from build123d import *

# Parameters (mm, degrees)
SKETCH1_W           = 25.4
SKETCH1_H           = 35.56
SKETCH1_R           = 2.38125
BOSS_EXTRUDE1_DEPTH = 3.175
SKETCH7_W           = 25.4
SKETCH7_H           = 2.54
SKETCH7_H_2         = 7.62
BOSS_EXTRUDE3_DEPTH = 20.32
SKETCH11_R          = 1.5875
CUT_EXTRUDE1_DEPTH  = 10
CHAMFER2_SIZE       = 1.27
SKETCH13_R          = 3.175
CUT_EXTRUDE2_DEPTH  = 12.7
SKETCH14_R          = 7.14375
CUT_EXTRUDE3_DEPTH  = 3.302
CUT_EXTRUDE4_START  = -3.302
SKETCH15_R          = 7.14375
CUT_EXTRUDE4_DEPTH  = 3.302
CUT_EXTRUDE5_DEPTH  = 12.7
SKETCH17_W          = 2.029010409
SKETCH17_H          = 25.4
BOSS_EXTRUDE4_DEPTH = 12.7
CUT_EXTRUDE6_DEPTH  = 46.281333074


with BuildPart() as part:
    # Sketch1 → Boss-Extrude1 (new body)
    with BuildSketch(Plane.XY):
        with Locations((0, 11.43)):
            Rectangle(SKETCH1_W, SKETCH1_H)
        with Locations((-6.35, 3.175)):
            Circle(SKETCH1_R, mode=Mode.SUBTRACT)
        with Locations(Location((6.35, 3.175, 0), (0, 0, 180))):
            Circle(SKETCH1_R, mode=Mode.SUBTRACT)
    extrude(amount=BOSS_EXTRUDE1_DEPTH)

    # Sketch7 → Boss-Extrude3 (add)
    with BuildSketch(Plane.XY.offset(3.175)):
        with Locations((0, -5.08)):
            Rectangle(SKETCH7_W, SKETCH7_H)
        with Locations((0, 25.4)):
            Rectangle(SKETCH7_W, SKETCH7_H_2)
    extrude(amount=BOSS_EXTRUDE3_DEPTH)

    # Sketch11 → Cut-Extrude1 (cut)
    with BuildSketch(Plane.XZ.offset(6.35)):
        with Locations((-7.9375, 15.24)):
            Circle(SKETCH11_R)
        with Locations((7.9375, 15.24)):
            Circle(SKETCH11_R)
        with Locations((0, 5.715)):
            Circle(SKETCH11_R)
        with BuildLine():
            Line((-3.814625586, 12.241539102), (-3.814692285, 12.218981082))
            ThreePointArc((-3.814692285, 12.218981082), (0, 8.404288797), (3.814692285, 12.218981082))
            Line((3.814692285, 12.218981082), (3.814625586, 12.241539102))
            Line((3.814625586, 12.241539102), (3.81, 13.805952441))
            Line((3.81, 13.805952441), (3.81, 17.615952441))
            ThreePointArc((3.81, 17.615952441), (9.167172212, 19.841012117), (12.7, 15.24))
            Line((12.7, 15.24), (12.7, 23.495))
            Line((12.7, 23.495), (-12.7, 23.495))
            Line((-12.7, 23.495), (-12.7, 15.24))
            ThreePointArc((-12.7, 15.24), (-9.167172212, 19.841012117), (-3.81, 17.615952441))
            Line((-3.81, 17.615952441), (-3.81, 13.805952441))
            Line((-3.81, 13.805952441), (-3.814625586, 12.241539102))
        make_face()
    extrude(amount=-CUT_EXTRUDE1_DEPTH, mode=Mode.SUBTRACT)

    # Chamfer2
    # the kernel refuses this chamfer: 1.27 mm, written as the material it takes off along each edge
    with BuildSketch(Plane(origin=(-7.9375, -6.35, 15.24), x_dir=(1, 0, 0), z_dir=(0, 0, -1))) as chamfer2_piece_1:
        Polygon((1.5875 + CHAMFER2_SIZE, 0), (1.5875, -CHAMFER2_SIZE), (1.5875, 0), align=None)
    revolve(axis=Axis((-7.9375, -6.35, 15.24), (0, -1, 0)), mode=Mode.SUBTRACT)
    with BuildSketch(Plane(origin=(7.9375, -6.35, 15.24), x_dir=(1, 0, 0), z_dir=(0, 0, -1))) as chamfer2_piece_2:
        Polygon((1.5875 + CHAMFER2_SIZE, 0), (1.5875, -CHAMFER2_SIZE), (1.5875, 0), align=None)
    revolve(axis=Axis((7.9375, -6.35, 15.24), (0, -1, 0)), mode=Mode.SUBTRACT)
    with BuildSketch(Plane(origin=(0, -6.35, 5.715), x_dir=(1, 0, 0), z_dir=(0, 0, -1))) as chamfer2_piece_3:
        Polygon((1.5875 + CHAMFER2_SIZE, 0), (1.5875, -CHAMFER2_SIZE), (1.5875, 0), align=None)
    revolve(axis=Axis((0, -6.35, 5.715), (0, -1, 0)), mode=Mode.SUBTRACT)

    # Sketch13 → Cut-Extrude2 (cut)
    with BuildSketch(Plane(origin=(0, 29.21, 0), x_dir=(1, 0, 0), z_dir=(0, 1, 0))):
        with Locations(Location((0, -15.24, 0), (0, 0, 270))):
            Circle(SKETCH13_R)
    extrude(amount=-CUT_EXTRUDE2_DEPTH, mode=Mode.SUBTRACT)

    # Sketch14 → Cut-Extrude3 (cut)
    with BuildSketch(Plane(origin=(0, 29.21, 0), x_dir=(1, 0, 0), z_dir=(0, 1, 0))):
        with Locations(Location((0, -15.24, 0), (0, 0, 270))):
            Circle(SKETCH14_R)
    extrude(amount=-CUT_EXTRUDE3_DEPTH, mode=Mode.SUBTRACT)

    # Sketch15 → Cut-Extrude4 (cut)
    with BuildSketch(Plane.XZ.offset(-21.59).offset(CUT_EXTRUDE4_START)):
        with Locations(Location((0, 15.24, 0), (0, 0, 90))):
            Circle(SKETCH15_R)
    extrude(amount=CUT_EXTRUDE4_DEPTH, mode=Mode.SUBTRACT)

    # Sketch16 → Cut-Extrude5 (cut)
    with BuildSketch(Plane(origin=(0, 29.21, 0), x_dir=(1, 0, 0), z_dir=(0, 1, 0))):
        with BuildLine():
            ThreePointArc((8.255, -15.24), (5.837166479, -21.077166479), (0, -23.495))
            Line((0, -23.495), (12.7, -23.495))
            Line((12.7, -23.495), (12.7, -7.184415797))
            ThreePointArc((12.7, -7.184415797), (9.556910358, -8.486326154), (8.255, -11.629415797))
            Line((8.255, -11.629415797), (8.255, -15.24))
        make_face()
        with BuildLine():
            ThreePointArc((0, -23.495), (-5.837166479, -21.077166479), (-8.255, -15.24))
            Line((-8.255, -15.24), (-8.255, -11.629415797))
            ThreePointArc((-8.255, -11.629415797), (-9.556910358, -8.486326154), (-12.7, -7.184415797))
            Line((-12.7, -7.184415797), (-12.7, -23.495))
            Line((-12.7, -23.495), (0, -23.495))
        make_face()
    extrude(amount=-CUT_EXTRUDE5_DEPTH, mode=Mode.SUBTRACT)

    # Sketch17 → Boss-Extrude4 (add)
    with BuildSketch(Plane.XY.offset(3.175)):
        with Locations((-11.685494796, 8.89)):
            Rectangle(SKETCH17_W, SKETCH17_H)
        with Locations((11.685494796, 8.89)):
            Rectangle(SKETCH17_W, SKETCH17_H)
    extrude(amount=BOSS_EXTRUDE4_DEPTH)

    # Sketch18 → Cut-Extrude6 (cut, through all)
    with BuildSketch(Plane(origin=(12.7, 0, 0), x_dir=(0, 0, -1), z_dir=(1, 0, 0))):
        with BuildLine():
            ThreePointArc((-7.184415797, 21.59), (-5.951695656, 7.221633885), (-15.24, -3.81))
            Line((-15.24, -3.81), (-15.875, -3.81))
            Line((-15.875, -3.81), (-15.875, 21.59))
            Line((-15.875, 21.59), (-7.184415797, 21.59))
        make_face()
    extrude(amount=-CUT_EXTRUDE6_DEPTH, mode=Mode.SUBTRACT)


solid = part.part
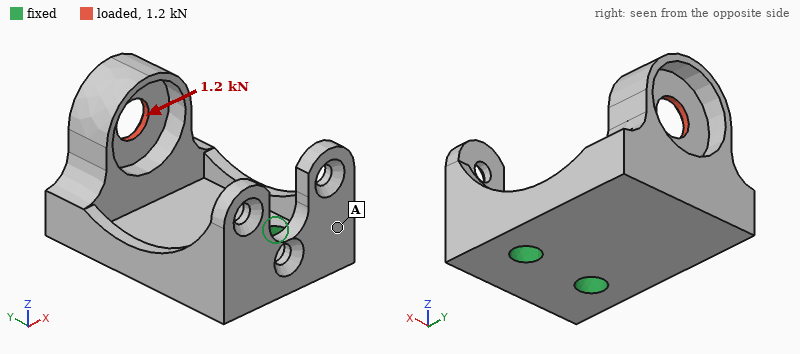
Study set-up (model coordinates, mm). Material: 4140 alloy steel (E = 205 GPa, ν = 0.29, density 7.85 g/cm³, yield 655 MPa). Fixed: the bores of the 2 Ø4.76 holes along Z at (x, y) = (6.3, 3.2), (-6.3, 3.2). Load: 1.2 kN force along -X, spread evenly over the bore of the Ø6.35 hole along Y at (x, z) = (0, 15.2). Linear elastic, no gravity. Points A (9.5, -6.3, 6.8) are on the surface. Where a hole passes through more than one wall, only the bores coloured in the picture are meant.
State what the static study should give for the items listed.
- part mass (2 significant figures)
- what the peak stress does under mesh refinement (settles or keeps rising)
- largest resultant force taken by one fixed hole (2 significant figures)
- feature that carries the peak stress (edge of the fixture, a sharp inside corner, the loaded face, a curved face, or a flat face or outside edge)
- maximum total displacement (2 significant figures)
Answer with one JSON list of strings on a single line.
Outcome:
["43 g", "keeps rising", "1.9 kN", "edge of the fixture", "0.13 mm"]
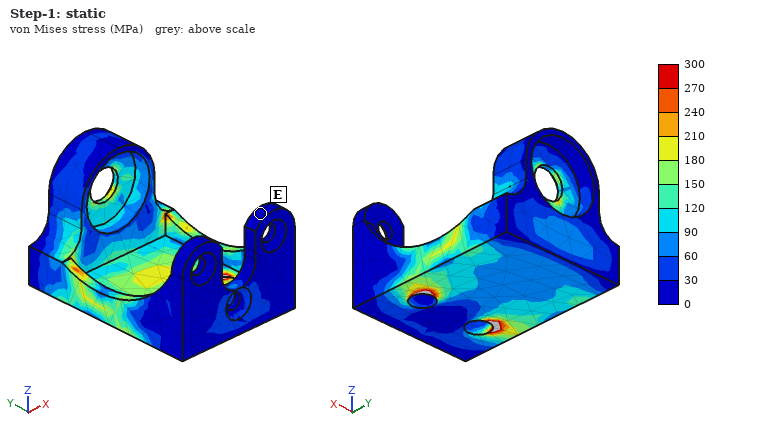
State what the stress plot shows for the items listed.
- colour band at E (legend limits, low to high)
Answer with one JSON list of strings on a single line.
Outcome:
["0 to 30 MPa"]
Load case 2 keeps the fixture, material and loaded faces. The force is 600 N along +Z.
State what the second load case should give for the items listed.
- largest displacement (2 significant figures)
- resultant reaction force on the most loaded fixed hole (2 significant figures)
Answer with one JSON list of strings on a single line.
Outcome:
["0.15 mm", "300 N"]
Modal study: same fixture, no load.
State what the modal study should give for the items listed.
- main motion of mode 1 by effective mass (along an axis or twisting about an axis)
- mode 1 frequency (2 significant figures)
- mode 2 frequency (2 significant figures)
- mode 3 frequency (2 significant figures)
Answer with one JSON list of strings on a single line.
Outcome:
["along Z", "2800 Hz", "5900 Hz", "10 kHz"]
